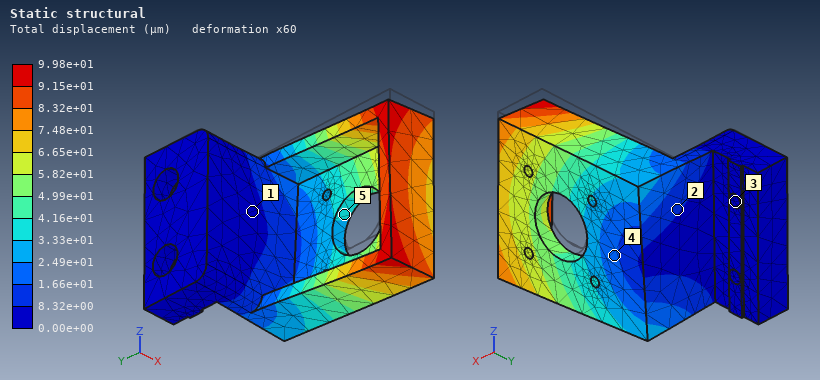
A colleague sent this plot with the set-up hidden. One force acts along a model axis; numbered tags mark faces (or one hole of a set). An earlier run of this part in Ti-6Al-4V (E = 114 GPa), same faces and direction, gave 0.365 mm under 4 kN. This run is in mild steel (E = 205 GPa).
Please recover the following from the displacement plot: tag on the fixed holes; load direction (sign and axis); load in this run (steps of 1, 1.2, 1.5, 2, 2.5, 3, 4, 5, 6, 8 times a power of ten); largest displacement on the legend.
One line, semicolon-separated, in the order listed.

3; -Z; 2 kN; 9.98e+01 µm
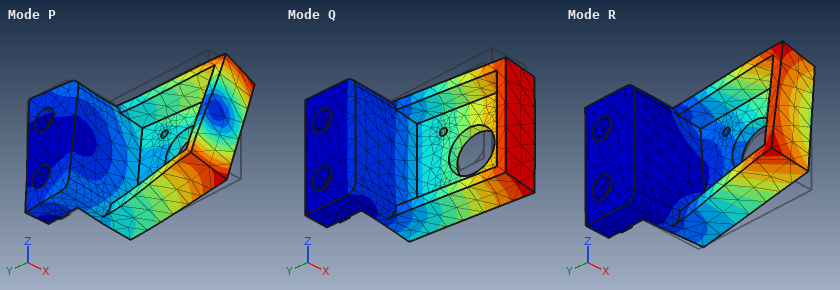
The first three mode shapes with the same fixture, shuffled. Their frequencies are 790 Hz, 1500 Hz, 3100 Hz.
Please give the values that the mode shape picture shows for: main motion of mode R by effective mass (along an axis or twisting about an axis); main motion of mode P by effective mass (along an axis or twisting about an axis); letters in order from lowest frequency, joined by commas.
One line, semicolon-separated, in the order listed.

along Z; along Z; Q, R, P
